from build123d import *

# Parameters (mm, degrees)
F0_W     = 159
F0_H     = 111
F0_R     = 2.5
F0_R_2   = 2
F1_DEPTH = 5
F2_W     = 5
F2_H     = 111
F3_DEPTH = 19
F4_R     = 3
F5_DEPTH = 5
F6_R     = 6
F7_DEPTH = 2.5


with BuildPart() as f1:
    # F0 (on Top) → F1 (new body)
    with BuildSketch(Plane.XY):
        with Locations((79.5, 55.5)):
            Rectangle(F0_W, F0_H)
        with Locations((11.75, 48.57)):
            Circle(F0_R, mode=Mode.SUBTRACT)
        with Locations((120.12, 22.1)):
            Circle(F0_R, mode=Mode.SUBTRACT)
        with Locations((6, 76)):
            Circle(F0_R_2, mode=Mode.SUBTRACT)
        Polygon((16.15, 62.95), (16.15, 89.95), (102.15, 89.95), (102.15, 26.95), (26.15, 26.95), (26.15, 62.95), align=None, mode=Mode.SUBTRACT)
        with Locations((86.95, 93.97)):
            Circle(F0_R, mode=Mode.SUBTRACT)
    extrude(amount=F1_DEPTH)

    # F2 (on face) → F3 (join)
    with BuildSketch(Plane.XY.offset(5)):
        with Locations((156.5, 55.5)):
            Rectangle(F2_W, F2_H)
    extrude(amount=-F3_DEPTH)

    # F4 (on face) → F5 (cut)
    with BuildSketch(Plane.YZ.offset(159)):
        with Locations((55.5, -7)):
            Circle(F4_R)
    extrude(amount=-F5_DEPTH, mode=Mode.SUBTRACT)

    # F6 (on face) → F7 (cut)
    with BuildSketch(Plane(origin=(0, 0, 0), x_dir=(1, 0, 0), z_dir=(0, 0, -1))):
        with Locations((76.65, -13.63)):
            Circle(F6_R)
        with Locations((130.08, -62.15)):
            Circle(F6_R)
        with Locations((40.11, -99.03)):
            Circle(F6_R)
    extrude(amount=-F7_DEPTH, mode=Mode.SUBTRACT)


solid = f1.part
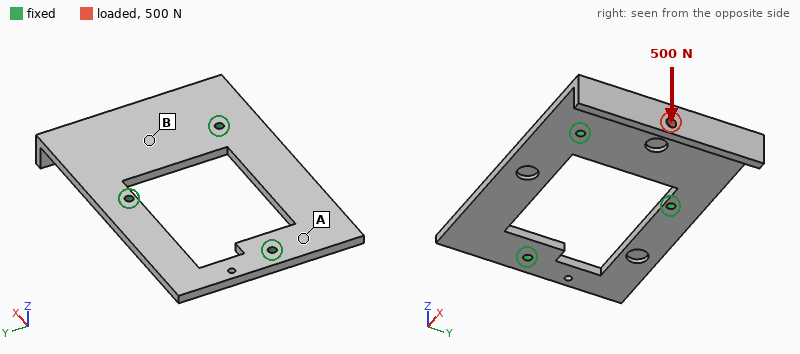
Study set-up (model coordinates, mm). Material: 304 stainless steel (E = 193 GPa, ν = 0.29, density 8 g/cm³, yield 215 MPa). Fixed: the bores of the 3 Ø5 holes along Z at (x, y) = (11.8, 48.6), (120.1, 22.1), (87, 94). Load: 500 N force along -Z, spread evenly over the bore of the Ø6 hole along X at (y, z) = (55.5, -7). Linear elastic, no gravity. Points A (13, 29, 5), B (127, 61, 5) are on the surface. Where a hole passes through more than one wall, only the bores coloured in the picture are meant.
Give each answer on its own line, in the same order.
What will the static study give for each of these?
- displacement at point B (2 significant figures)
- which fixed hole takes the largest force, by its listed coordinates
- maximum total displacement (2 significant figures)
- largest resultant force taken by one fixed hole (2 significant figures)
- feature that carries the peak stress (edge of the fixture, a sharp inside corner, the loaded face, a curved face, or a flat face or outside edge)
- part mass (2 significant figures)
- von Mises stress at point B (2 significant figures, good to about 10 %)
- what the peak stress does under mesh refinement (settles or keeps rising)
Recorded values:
0.048 mm
(120.1, 22.1)
0.23 mm
410 N
edge of the fixture
560 g
20 MPa
keeps rising
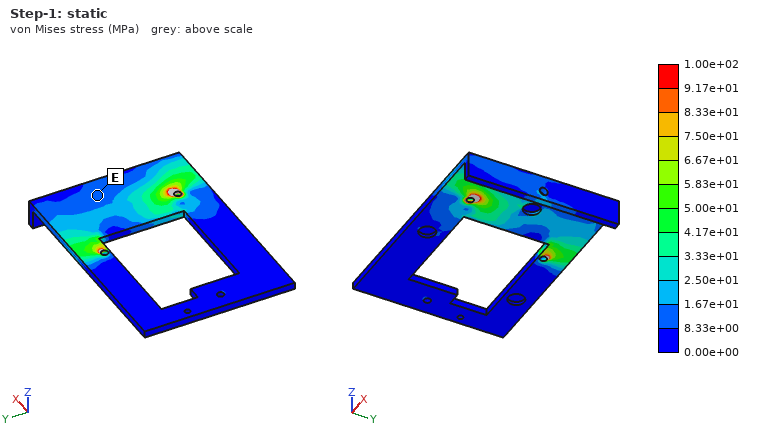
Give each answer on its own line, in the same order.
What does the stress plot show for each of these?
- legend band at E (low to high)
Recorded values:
8.33e+00 to 1.67e+01 MPa
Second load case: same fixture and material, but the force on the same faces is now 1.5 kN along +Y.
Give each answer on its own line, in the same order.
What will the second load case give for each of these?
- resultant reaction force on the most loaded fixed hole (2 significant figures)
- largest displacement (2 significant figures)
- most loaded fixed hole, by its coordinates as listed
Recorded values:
1.6 kN
0.13 mm
(120.1, 22.1)
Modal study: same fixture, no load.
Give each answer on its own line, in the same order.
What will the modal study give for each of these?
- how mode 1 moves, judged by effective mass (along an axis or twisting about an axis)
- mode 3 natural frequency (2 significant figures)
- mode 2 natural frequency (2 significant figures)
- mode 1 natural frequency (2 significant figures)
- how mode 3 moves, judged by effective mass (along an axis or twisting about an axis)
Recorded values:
along Z
1300 Hz
1200 Hz
730 Hz
along Z
